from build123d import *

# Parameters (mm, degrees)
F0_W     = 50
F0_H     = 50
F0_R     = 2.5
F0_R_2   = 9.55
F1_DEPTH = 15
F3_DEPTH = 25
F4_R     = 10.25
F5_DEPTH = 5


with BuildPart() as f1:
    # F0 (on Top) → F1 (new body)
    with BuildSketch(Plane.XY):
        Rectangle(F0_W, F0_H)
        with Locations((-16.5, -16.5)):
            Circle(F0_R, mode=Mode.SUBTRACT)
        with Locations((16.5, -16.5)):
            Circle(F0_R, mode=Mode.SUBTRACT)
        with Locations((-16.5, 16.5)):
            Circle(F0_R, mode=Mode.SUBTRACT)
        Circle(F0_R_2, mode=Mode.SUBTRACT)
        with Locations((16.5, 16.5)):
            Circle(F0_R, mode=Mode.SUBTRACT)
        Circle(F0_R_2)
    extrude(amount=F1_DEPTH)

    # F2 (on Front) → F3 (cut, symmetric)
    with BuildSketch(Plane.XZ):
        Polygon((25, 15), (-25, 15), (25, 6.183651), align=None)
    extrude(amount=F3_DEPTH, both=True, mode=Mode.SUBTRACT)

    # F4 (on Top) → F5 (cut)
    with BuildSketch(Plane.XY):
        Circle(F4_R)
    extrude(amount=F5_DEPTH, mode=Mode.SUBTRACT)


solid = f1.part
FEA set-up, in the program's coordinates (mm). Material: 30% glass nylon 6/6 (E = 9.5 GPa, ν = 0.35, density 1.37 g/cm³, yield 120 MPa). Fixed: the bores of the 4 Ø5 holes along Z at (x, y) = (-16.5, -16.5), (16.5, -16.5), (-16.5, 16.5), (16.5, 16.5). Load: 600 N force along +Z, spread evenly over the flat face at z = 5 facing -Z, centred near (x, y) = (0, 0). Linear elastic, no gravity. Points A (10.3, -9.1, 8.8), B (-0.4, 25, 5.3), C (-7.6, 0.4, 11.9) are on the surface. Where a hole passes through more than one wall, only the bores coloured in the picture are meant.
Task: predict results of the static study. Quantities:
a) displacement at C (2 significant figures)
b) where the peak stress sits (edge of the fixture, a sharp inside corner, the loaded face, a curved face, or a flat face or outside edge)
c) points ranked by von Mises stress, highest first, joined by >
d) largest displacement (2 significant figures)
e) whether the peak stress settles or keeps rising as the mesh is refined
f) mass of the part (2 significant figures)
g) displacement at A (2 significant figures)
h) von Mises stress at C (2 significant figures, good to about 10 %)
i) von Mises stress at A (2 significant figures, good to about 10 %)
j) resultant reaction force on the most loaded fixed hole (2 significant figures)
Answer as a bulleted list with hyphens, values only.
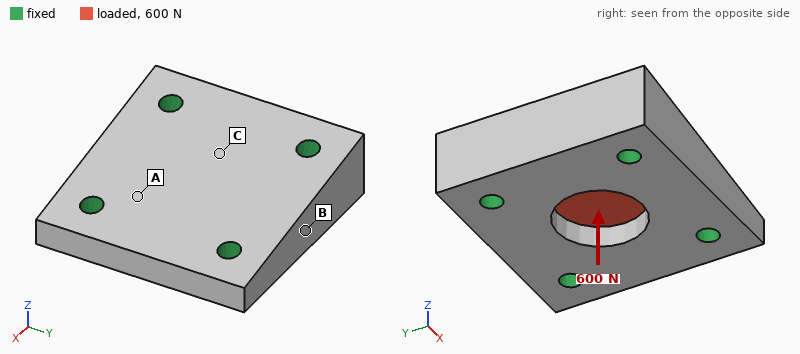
- 10.0 µm
- edge of the fixture
- C > A > B
- 18 µm
- keeps rising
- 33 g
- 7.5 µm
- 3.0 MPa
- 1.6 MPa
- 180 N
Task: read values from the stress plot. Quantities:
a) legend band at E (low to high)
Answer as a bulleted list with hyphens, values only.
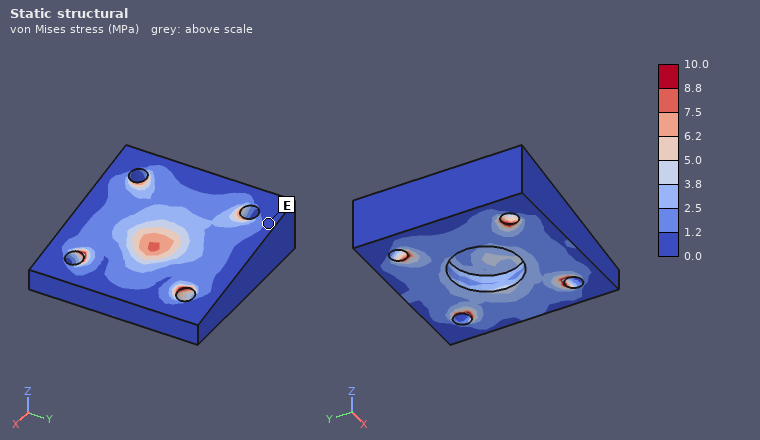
- 0.0 to 1.2 MPa
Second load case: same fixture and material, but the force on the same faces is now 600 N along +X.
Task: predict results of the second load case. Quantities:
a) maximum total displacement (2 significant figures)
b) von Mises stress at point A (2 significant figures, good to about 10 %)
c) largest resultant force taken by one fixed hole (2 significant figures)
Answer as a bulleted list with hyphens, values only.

- 6.8 µm
- 2.0 MPa
- 200 N
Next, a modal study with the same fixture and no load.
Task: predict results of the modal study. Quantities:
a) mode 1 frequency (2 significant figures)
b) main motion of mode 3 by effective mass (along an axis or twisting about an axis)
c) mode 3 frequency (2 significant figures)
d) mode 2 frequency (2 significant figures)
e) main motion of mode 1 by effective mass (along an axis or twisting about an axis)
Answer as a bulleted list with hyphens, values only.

- 14 kHz
- twisting about X
- 18 kHz
- 16 kHz
- along Z
